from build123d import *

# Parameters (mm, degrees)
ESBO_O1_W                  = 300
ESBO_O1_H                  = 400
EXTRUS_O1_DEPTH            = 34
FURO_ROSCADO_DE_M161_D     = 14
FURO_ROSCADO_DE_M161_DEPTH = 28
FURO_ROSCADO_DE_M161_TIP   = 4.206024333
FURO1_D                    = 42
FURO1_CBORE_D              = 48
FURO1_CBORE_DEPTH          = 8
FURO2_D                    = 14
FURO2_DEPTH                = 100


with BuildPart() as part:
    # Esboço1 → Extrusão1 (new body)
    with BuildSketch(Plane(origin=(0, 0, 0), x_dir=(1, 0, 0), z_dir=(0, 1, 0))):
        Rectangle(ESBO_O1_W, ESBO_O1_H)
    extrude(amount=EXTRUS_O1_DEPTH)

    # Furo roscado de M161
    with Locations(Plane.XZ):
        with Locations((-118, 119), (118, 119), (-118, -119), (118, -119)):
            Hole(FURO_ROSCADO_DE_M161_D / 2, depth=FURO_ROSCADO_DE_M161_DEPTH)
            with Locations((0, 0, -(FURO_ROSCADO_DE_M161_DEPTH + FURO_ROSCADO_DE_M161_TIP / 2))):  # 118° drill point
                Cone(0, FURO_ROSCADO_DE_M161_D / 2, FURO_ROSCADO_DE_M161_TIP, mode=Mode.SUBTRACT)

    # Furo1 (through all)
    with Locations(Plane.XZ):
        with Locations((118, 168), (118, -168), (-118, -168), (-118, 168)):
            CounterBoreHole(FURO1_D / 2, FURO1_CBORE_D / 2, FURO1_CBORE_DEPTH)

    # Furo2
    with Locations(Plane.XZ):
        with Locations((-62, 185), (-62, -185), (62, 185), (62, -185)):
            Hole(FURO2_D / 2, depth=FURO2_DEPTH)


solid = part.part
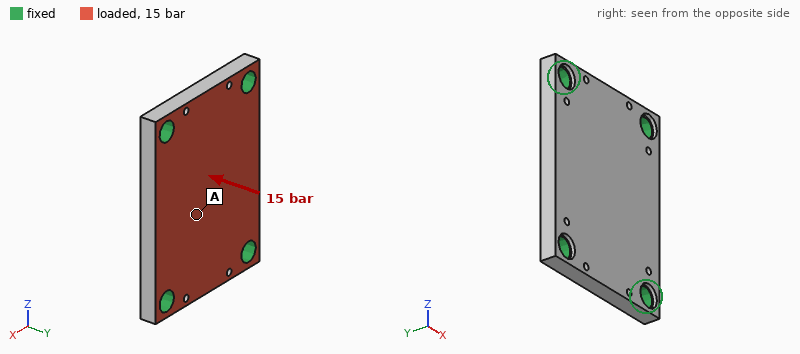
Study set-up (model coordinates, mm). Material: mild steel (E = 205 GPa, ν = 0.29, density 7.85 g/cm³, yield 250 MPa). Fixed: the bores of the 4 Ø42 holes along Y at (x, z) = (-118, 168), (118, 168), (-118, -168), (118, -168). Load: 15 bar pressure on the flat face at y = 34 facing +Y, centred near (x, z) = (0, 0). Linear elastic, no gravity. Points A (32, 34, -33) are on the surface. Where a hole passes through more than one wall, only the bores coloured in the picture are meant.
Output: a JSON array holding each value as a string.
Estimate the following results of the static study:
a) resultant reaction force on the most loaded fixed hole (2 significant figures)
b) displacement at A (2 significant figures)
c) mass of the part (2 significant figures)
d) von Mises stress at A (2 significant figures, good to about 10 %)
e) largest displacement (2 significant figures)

["44 kN", "0.10 mm", "30 kg", "30 MPa", "0.11 mm"]
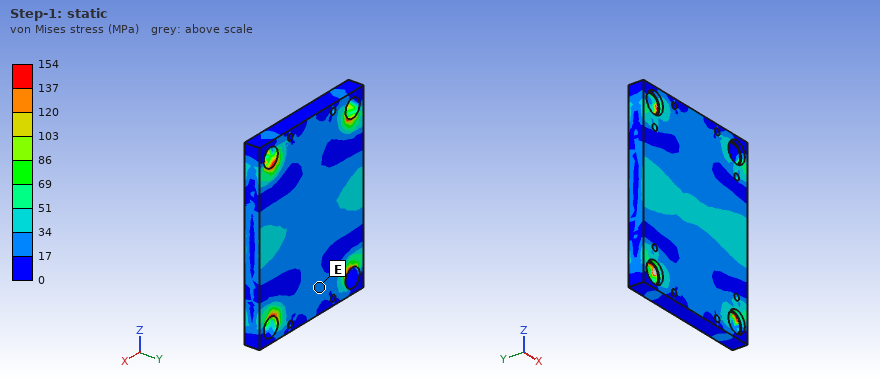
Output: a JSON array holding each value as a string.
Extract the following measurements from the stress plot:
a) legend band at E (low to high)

["17 to 34 MPa"]
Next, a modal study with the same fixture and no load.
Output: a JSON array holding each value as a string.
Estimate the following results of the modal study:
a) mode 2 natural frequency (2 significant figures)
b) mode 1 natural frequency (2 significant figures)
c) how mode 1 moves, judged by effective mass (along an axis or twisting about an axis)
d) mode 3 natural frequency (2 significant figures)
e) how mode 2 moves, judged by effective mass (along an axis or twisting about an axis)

["1900 Hz", "1300 Hz", "along Y", "2800 Hz", "twisting about Z"]
